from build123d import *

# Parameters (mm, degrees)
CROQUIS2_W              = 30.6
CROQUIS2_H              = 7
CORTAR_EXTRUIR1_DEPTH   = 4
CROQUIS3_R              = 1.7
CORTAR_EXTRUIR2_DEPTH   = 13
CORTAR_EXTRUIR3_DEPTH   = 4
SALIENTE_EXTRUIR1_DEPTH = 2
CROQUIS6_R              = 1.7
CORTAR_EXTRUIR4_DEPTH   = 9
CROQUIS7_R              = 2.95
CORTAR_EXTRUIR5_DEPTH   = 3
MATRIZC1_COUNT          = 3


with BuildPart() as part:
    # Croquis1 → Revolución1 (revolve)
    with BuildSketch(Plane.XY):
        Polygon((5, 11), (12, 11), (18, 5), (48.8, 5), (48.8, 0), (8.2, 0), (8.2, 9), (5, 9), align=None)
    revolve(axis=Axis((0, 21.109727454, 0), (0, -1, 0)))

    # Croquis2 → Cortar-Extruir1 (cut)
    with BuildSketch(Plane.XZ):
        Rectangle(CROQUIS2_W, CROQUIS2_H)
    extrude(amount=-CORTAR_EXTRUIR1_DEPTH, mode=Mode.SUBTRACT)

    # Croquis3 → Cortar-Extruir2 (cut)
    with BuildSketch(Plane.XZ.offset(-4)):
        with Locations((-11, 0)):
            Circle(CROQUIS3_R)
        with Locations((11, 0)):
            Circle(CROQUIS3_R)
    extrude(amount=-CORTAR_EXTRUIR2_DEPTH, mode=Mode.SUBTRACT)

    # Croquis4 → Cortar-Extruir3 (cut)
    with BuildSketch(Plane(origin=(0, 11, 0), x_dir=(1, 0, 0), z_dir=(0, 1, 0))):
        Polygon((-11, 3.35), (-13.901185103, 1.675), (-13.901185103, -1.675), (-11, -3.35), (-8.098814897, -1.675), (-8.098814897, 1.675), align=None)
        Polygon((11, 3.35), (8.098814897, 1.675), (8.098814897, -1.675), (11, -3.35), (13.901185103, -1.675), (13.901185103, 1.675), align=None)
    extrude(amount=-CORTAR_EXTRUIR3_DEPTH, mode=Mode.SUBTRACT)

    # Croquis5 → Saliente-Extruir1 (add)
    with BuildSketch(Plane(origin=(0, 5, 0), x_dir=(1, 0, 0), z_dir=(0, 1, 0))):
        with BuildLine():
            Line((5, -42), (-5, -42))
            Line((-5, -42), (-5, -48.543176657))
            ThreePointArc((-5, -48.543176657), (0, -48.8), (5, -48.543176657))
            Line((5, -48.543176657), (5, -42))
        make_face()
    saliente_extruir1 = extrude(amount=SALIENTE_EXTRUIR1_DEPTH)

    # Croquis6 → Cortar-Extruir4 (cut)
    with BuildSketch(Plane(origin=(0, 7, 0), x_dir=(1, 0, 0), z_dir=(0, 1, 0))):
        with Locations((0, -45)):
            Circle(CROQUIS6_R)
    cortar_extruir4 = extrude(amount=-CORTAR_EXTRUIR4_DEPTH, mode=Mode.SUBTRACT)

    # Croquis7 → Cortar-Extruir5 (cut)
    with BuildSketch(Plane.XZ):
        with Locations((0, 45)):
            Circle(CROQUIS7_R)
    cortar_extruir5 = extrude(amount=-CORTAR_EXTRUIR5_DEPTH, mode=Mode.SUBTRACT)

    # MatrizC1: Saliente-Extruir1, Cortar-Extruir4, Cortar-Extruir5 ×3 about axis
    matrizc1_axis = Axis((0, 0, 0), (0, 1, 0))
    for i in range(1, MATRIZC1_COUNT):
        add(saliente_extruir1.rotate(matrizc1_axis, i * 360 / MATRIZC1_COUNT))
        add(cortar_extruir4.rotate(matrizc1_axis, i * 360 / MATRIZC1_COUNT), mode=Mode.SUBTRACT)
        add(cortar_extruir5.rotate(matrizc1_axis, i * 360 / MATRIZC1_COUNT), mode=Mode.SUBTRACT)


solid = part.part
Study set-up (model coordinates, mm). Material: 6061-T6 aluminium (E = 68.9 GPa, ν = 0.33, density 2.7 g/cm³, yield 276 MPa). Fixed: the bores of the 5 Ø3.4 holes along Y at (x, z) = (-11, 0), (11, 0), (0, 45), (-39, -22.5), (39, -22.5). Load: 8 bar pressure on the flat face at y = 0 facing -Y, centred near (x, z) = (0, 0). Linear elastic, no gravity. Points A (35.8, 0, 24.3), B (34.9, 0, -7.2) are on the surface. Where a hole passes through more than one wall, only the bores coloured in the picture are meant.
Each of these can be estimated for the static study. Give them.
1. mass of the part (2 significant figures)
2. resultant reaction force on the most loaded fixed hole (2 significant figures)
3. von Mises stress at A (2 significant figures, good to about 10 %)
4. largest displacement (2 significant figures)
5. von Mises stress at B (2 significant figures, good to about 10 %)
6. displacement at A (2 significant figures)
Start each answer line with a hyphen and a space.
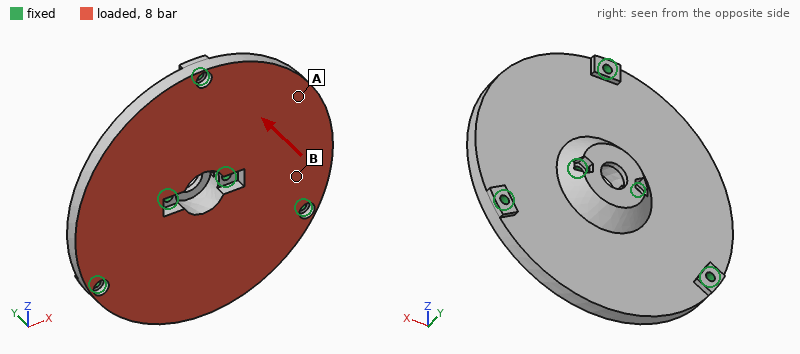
- 110 g
- 1.5 kN
- 18 MPa
- 0.17 mm
- 43 MPa
- 0.11 mm
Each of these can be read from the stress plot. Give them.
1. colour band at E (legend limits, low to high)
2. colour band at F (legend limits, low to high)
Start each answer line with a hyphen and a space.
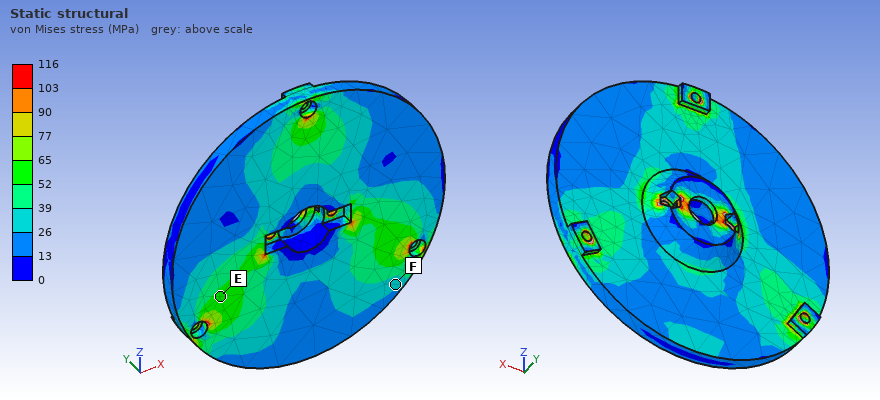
- 52 to 65 MPa
- 26 to 39 MPa
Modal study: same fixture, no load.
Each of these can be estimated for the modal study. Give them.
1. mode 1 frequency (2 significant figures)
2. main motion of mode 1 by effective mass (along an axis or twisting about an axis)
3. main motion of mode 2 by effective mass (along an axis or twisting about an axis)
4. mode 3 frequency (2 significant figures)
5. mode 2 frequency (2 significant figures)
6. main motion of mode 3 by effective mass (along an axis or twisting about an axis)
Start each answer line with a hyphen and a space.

- 3100 Hz
- twisting about X
- twisting about Z
- 4400 Hz
- 3600 Hz
- along Y
